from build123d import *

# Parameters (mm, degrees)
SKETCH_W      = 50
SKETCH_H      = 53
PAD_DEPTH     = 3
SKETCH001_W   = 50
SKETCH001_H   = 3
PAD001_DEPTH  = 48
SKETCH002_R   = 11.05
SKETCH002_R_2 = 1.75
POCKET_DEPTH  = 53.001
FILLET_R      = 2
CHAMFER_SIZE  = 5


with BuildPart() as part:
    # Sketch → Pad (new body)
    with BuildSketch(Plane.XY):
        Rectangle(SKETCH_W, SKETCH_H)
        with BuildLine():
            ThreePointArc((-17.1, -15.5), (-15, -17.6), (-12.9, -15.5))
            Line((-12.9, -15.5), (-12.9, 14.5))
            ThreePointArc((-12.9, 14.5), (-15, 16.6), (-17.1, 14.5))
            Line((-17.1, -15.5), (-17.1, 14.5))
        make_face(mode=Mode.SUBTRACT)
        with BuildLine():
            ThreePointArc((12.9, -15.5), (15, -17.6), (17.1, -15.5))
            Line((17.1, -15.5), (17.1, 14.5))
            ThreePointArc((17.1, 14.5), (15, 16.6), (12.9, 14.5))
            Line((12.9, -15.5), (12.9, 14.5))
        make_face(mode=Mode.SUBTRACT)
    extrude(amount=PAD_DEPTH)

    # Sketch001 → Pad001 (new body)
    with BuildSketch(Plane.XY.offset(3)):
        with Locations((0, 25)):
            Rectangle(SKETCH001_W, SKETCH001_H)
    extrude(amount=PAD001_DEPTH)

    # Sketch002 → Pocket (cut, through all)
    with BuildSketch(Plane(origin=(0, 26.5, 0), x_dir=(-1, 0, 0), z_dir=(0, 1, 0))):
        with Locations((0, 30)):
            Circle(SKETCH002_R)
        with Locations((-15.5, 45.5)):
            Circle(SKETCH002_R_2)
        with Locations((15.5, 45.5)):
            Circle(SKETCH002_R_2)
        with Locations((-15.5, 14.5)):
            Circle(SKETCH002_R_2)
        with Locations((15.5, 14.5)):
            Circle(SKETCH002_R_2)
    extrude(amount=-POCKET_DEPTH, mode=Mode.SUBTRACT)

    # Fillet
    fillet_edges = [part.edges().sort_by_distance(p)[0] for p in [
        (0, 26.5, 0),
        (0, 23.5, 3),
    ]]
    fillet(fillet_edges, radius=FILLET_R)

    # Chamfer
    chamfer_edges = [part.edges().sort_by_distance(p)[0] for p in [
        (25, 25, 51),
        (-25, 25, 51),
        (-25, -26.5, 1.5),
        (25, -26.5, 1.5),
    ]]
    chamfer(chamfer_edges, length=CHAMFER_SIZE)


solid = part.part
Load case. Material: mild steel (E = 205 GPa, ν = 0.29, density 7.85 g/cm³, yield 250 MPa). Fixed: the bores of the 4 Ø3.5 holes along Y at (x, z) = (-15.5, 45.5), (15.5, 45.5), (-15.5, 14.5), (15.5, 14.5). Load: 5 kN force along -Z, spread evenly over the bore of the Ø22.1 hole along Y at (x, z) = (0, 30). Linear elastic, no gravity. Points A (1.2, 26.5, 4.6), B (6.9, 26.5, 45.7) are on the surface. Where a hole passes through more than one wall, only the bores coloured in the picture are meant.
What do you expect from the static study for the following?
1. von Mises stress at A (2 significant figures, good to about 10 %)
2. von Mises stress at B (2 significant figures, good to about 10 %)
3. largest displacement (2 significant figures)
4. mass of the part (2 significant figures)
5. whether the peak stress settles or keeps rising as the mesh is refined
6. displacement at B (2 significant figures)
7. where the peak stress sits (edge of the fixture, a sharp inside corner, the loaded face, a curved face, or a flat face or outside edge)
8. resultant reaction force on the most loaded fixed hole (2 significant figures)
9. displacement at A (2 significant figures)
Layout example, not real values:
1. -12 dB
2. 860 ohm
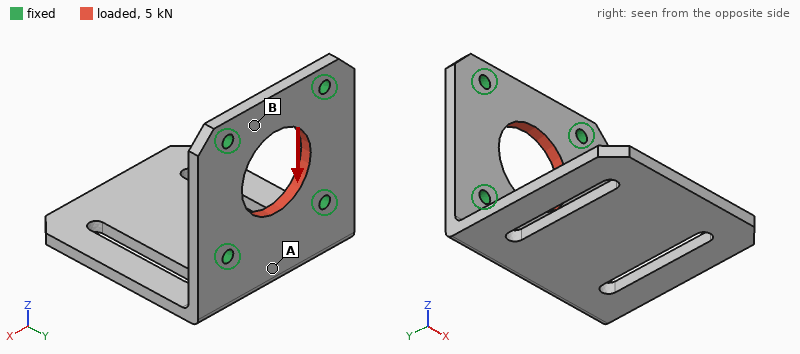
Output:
1. 9.7 MPa
2. 31 MPa
3. 5.0 µm
4. 100 g
5. keeps rising
6. 3.2 µm
7. edge of the fixture
8. 1.3 kN
9. 1.9 µm
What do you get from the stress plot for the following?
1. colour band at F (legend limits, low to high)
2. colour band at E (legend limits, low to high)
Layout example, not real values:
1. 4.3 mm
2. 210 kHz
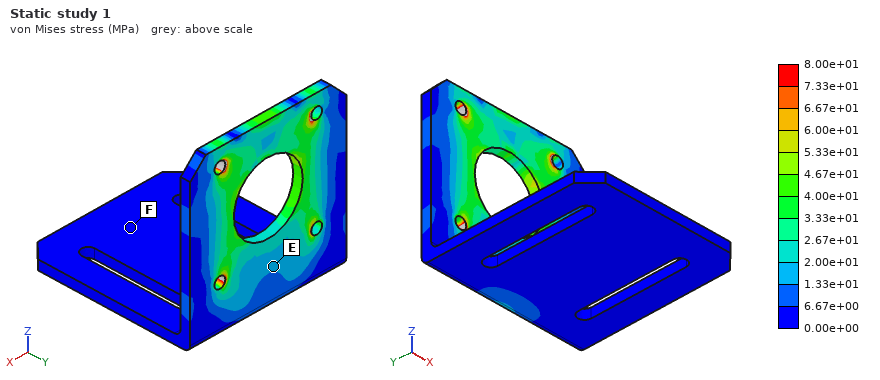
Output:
1. 0.00e+00 to 6.67e+00 MPa
2. 1.33e+01 to 2.00e+01 MPa
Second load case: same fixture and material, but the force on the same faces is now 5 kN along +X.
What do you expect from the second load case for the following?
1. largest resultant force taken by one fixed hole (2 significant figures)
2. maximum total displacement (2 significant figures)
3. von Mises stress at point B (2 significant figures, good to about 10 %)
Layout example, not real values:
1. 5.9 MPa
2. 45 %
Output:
1. 1.3 kN
2. 3.8 µm
3. 24 MPa
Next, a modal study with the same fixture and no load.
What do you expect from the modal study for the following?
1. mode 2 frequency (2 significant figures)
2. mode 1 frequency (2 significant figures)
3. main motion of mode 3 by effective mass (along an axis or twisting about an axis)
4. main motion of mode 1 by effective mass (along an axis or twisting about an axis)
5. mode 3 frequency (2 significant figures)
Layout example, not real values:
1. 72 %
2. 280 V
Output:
1. 1900 Hz
2. 710 Hz
3. along X
4. along Z
5. 2700 Hz
